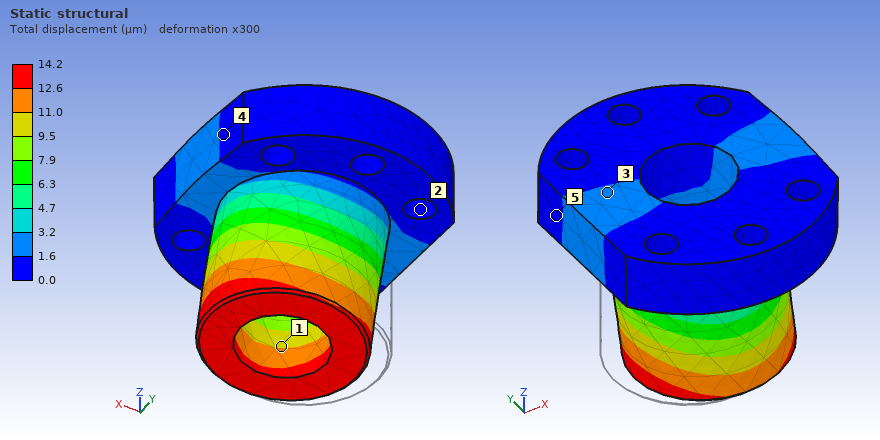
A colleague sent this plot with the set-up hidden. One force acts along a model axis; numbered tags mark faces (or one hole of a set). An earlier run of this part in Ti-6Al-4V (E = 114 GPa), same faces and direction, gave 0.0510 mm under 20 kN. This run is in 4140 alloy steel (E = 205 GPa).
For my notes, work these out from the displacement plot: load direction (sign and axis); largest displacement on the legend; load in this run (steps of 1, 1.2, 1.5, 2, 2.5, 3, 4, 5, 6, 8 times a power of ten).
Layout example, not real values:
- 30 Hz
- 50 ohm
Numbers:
- +X
- 14.2 µm
- 10 kN
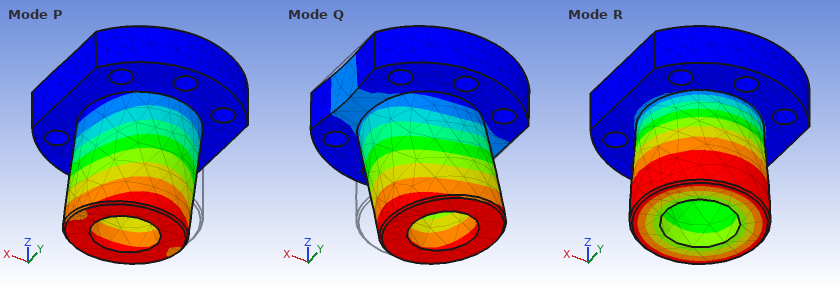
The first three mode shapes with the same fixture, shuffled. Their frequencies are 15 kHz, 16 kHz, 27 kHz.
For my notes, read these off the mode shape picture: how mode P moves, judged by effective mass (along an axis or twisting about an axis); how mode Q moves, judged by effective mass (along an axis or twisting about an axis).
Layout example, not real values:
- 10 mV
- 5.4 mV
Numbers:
- along Y
- along X
